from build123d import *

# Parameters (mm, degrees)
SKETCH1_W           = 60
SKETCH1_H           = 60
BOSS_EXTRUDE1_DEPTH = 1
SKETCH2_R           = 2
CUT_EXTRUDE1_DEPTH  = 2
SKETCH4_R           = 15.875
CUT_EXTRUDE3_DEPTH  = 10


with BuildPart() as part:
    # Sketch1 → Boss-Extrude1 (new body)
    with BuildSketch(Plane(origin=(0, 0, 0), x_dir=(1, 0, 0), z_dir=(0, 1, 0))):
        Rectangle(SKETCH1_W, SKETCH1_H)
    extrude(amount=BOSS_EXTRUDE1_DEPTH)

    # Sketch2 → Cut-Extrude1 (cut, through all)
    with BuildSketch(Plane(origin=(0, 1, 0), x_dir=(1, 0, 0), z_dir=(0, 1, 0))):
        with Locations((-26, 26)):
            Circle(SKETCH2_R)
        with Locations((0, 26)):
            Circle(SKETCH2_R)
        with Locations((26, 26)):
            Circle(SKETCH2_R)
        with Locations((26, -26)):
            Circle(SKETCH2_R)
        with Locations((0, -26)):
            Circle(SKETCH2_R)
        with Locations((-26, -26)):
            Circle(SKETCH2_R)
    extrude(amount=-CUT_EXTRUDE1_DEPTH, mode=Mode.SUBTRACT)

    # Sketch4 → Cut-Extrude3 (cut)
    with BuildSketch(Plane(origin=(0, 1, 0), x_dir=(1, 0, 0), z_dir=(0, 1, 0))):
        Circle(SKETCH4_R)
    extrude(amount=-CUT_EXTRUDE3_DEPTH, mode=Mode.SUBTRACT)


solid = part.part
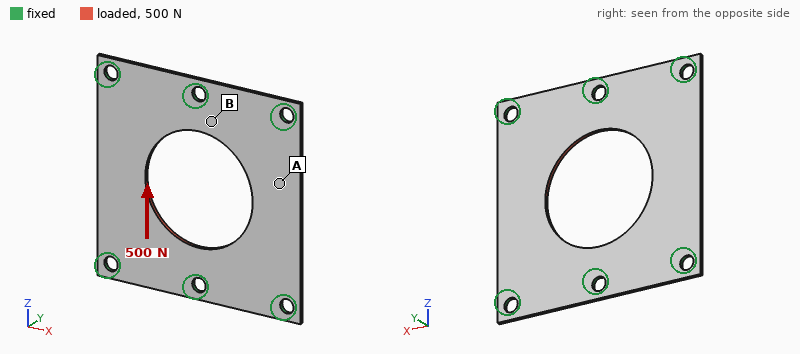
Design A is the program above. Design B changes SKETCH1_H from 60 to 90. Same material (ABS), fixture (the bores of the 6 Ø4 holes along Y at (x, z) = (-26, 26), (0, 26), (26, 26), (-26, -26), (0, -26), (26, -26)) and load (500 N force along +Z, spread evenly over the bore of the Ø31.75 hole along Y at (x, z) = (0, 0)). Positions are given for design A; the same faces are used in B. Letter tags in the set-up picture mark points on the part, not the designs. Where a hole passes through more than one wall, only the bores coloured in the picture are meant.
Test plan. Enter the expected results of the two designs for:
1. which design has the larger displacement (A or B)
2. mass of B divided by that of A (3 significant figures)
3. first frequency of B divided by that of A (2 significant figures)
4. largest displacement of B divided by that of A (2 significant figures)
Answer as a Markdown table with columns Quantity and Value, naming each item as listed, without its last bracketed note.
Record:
| Quantity | Value |
|---|---|
| which design has the larger displacement | A |
| mass of B divided by that of A | 1.66 |
| first frequency of B divided by that of A | 0.97 |
| largest displacement of B divided by that of A | 0.92 |
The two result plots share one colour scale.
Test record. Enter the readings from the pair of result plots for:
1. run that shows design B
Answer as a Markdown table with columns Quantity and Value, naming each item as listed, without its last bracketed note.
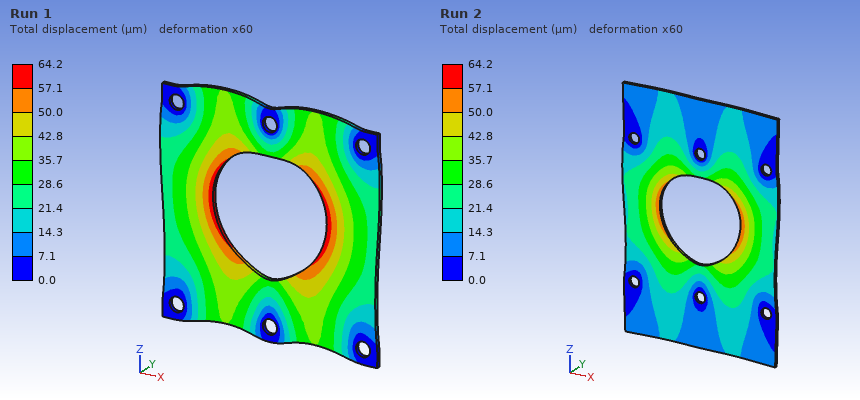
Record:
| Quantity | Value |
|---|---|
| run that shows design B | Run 2 |
